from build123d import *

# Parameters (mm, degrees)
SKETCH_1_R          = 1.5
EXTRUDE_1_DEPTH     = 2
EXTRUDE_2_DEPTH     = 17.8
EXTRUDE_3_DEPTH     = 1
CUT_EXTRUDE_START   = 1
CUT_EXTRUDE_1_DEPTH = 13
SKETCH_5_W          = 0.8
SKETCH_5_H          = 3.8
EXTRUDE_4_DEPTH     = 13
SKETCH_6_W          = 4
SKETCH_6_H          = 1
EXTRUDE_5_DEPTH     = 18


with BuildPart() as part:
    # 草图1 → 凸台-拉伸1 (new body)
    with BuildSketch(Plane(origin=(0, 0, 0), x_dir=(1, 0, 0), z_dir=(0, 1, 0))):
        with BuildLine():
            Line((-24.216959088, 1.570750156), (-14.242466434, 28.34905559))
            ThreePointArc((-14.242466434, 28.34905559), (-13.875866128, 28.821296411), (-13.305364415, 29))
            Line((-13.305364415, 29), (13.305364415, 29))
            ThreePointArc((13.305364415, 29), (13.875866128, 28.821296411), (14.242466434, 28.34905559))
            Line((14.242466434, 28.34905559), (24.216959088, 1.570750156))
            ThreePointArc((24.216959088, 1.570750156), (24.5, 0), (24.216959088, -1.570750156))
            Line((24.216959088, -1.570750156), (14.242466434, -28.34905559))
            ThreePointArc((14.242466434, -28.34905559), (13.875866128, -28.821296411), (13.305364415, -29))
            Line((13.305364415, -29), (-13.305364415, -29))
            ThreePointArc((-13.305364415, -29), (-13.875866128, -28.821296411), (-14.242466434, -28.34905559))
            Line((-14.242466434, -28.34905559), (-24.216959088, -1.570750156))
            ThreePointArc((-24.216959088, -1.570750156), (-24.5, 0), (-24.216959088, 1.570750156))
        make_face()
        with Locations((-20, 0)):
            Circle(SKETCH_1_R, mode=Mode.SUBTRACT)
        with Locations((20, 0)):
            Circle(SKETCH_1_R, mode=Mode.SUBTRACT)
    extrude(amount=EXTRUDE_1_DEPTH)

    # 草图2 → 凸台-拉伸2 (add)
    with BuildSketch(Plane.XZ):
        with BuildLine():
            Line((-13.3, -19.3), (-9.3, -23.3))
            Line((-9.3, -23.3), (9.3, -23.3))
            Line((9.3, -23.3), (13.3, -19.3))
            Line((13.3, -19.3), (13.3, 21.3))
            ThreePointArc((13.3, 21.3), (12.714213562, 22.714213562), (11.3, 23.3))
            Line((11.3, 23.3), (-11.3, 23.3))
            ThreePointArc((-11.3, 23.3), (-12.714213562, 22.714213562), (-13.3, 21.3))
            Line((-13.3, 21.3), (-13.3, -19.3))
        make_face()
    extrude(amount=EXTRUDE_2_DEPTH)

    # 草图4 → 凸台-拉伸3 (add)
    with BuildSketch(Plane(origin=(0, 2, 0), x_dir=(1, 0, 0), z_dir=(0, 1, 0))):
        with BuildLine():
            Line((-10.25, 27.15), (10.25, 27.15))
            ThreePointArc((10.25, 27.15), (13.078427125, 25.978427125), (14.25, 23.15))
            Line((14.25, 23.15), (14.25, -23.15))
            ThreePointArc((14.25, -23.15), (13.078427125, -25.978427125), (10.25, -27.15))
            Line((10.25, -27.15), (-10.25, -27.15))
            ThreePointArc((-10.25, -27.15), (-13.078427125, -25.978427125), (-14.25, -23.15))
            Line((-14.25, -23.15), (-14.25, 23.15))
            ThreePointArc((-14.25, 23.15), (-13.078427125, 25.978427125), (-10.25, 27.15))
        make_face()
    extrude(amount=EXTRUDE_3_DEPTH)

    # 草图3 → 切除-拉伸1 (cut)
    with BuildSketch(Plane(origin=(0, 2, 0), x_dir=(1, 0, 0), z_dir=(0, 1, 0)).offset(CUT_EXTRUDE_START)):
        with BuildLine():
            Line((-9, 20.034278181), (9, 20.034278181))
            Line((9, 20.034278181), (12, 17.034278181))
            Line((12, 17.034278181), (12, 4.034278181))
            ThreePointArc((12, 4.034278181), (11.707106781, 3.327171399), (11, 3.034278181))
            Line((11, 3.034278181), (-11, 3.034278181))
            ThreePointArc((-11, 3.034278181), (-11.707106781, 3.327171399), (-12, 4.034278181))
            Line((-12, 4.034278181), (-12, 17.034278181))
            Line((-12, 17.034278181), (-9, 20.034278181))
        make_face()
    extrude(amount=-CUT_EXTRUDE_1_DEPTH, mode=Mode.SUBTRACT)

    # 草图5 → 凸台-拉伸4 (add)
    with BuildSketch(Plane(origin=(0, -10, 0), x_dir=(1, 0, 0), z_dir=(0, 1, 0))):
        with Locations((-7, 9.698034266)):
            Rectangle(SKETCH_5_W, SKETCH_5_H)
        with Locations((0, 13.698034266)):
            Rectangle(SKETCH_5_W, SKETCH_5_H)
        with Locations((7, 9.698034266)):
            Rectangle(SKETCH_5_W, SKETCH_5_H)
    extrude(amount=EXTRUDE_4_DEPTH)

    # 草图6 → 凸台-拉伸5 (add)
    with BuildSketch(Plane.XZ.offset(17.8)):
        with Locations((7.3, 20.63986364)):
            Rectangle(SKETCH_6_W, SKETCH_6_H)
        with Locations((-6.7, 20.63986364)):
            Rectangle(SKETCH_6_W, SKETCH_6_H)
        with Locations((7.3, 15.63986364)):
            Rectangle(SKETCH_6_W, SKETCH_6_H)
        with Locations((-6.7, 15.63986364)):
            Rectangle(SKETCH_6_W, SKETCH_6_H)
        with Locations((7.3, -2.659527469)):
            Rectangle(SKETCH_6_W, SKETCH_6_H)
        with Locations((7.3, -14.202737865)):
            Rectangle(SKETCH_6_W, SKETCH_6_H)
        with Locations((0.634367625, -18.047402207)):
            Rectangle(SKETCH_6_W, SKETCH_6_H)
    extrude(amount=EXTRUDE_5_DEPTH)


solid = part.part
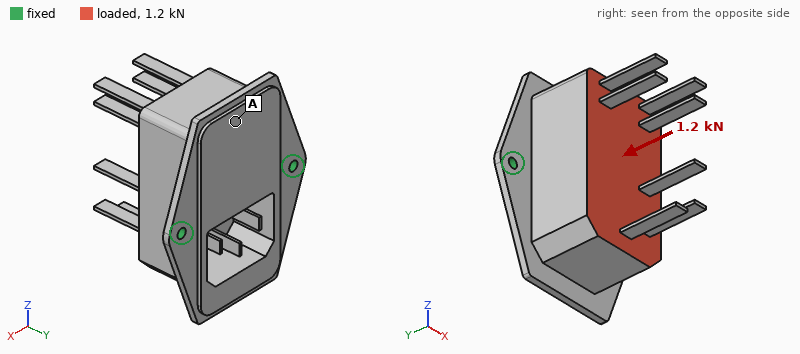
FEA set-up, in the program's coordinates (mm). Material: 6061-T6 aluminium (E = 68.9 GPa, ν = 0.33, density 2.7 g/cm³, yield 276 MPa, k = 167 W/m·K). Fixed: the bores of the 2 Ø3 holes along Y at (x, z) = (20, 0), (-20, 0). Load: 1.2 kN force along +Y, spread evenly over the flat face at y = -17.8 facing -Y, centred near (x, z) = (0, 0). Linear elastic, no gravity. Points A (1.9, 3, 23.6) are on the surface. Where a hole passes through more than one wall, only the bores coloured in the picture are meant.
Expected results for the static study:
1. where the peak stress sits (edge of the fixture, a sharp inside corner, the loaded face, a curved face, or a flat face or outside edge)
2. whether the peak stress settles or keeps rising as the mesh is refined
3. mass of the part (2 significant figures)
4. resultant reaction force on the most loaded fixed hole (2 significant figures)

edge of the fixture
keeps rising
63 g
620 N
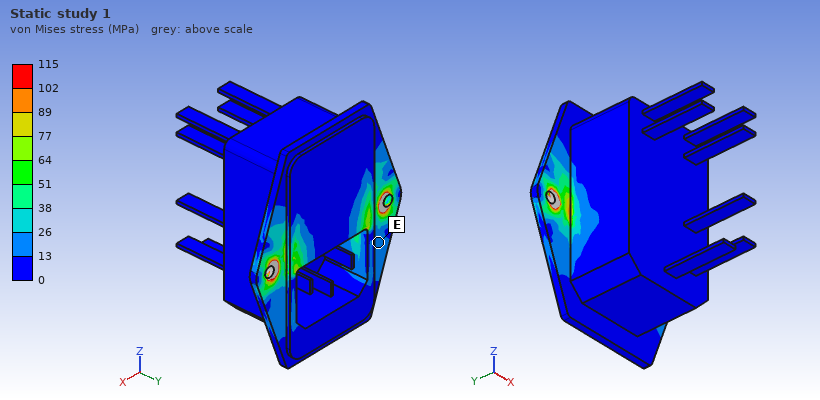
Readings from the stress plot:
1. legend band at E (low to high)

13 to 26 MPa
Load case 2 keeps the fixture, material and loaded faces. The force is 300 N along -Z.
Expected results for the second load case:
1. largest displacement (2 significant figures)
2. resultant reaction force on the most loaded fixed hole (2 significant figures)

0.43 mm
160 N
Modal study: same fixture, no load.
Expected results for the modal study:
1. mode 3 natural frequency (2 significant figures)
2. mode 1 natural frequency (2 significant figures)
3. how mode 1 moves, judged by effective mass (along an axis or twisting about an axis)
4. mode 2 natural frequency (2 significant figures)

2500 Hz
830 Hz
along Z
2500 Hz
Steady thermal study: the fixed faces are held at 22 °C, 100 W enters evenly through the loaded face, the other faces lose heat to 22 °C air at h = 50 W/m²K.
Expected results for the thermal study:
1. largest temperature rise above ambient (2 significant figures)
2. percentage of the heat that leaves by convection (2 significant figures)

72 K
26 %
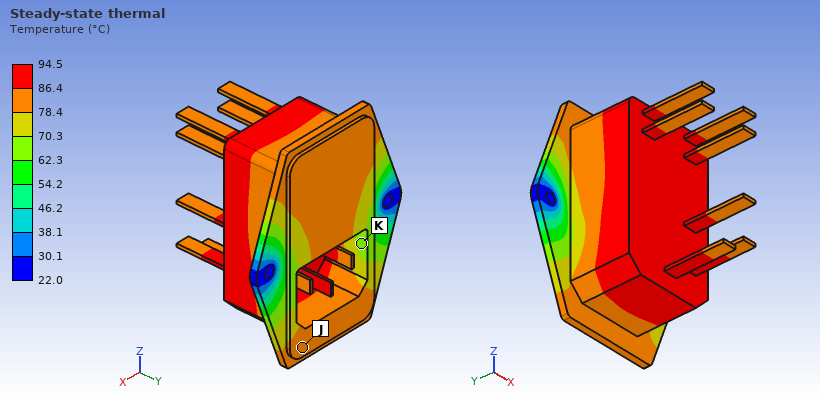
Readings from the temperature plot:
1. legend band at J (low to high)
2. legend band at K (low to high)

78.4 to 86.4 °C
62.3 to 70.3 °C
